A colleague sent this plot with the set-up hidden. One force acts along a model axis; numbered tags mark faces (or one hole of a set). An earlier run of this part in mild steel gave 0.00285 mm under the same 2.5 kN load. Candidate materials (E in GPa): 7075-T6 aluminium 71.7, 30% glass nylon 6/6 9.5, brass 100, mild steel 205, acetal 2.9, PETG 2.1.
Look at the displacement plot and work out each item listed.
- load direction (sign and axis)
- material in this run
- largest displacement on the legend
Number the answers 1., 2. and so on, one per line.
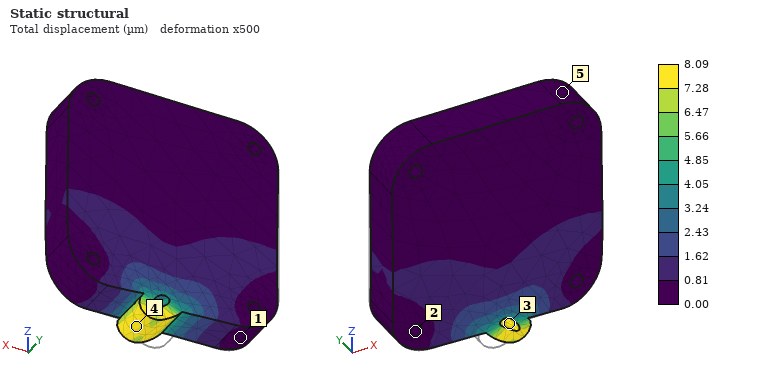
1. +X
2. 7075-T6 aluminium
3. 8.09 µm
